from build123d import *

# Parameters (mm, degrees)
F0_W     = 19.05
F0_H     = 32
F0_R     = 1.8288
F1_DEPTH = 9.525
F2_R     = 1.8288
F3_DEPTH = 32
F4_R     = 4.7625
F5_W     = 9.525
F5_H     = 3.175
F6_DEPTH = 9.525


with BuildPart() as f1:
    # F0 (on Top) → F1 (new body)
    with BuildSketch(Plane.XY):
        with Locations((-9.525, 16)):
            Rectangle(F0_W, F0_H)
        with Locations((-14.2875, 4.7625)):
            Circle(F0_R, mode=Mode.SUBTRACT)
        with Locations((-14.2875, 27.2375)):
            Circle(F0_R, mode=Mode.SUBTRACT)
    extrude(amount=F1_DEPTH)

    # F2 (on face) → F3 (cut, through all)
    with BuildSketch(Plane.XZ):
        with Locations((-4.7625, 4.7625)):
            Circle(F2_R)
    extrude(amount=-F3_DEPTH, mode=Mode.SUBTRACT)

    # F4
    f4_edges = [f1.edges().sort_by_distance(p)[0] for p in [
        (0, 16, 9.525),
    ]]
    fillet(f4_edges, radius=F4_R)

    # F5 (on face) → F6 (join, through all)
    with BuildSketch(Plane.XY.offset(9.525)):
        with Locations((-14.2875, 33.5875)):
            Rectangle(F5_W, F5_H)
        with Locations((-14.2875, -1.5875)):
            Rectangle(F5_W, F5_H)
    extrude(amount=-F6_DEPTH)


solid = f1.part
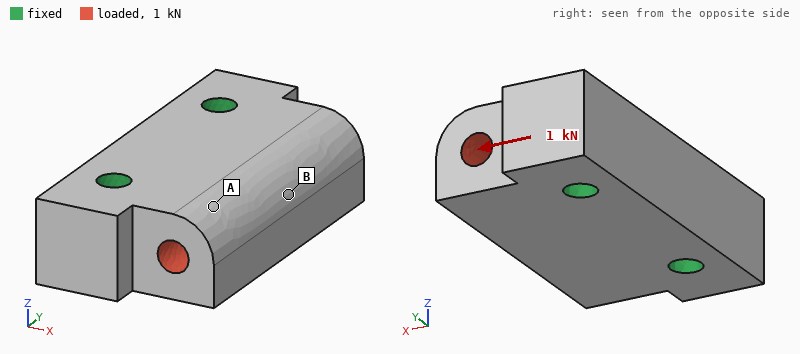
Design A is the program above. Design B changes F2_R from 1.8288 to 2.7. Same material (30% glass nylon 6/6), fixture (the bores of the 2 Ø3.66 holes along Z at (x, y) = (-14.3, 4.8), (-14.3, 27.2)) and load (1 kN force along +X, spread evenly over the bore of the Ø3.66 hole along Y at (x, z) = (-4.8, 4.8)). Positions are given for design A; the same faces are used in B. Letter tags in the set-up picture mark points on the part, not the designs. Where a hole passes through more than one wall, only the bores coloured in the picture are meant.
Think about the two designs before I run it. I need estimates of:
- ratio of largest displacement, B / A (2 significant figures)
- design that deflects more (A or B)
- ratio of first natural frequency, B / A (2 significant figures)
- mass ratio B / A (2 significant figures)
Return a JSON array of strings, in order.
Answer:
["1.3", "B", "0.98", "0.93"]
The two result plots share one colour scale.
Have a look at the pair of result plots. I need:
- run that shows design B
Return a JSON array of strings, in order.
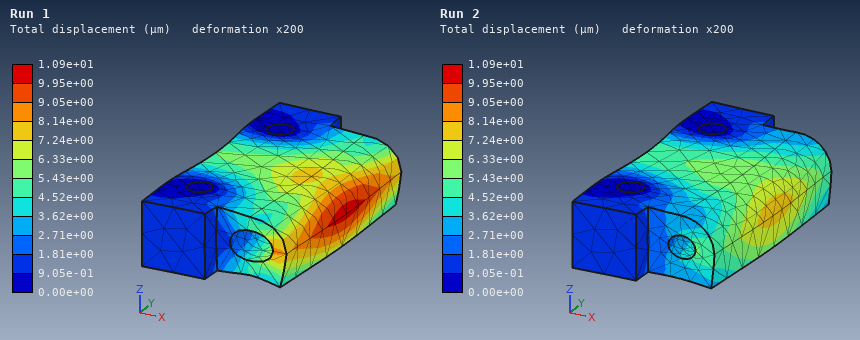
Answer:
["Run 1"]
